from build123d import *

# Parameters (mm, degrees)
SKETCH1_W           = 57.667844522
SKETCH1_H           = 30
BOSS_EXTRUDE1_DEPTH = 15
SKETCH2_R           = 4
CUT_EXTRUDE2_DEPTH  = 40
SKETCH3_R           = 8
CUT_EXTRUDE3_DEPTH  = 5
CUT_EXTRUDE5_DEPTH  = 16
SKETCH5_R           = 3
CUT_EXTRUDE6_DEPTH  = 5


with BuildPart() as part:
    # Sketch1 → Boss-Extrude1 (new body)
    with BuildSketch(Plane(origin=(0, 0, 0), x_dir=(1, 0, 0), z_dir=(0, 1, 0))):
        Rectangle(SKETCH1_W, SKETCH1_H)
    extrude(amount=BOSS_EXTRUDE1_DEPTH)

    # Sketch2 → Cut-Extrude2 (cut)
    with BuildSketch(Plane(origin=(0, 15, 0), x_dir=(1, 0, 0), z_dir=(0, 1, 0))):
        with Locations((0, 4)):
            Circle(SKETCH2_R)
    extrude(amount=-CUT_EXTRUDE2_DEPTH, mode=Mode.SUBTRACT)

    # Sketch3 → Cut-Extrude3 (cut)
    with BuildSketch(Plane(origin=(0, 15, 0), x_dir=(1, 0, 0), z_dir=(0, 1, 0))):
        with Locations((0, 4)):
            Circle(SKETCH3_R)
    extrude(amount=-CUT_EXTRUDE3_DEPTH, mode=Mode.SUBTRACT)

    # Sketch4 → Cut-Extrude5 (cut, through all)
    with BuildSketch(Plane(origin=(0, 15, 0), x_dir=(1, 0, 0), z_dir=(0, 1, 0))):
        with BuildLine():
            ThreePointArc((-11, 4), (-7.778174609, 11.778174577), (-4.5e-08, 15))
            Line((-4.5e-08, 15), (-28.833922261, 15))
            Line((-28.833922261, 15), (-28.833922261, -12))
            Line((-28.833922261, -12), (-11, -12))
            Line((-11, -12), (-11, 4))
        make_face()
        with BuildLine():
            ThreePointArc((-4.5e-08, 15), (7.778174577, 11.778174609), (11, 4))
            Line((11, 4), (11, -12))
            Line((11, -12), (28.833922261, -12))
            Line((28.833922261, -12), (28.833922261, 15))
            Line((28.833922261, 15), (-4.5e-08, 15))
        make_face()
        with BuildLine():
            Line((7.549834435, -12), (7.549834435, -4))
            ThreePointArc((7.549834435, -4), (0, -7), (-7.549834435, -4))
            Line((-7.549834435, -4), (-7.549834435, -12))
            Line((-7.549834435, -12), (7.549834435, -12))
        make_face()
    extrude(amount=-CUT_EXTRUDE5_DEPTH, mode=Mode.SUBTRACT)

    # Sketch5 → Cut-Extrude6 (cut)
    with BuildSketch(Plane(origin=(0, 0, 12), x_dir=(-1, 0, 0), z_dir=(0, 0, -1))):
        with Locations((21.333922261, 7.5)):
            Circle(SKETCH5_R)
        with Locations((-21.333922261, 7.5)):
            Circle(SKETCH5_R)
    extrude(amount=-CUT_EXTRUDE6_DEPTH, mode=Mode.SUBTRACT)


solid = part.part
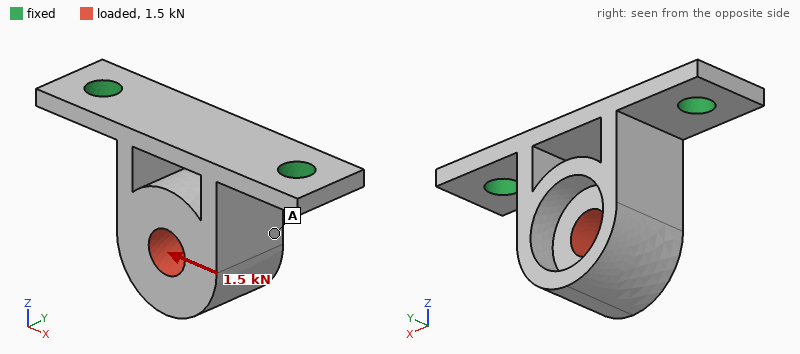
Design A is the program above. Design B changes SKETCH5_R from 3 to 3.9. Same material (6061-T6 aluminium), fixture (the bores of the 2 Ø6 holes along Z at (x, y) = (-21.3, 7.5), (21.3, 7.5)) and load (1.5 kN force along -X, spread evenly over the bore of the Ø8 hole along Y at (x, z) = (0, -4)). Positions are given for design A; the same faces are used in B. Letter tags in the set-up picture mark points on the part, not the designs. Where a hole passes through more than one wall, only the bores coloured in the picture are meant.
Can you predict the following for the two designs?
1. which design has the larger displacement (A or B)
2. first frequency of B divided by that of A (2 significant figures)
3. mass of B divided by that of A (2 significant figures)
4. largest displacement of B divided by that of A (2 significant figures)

A
1.1
0.98
0.86
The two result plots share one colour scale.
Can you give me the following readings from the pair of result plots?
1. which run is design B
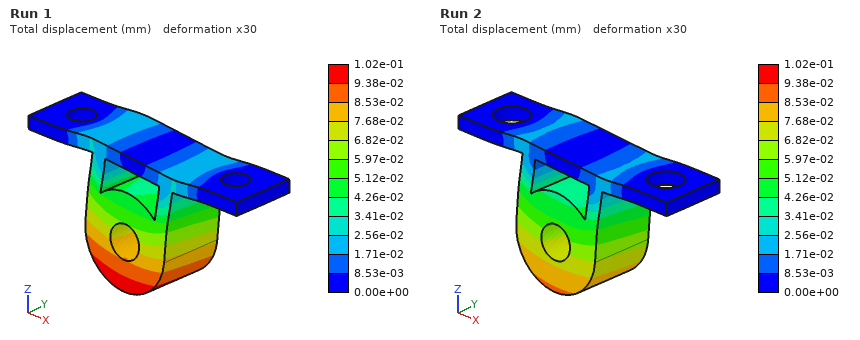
Run 2
